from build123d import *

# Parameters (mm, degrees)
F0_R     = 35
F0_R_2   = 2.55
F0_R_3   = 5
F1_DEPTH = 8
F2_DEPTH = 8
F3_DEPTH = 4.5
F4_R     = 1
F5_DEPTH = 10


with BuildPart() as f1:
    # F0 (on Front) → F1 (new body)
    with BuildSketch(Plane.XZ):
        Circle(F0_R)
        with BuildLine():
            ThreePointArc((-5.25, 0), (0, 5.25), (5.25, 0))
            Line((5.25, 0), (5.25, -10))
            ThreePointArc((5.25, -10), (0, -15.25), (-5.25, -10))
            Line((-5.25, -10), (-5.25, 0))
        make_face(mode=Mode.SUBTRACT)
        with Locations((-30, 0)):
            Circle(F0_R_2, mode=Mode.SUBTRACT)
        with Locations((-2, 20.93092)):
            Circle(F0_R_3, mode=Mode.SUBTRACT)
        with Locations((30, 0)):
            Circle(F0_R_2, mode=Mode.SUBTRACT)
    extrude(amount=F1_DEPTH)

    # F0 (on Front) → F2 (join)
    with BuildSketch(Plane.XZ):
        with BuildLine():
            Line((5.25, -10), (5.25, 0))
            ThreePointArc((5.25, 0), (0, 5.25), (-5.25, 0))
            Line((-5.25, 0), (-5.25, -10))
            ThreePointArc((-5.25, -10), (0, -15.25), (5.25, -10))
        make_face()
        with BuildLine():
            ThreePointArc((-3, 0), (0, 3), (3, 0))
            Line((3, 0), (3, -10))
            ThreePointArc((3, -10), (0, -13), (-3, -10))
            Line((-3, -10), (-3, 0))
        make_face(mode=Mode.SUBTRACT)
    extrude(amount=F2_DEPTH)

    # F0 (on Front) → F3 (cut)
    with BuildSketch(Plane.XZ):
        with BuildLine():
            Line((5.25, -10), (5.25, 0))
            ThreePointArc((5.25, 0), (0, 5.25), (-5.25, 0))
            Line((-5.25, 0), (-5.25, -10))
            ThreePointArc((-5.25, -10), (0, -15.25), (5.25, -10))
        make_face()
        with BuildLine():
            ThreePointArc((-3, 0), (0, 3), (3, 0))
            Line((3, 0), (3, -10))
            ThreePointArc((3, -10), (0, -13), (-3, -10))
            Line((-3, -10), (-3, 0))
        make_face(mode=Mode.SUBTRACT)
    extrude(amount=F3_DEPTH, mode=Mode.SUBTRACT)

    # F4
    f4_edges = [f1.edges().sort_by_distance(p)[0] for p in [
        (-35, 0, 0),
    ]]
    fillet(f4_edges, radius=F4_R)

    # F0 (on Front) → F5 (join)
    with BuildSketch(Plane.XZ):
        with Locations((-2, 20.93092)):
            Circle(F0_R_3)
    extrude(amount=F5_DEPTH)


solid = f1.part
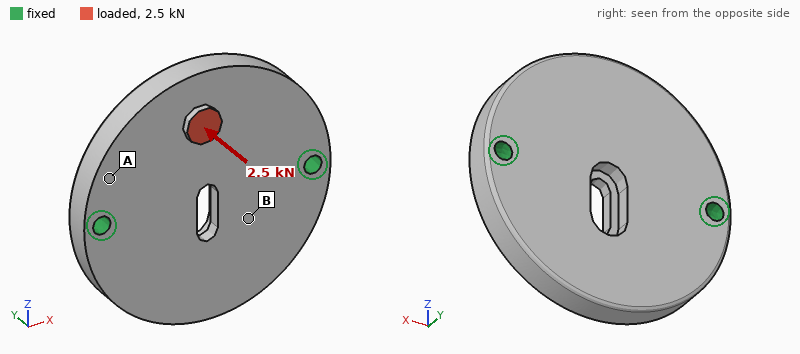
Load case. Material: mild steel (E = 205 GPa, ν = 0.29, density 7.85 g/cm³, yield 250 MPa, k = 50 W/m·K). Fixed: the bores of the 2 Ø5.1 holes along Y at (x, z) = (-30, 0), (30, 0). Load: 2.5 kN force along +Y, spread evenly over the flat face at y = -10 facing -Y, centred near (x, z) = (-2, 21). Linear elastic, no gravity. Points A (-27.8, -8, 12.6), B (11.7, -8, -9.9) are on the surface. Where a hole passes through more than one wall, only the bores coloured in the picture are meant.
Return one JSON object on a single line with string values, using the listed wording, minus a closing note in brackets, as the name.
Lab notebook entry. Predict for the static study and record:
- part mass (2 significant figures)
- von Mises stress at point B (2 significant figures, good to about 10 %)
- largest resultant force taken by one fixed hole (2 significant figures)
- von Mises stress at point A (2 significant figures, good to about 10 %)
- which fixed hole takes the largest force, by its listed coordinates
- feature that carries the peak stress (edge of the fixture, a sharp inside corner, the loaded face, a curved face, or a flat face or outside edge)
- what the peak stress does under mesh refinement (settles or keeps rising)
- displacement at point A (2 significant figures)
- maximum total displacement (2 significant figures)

{"part mass": "230 g", "von Mises stress at point B": "23 MPa", "largest resultant force taken by one fixed hole": "1.4 kN", "von Mises stress at point A": "61 MPa", "which fixed hole takes the largest force, by its listed coordinates": "(-30, 0)", "feature that carries the peak stress": "edge of the fixture", "what the peak stress does under mesh refinement": "keeps rising", "displacement at point A": "13 µm", "maximum total displacement": "69 µm"}
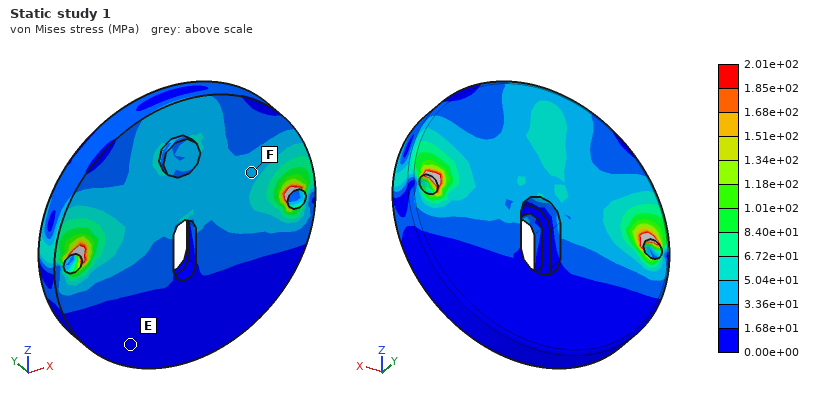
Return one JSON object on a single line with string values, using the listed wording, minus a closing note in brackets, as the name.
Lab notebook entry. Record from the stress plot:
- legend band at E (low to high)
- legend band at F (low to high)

{"legend band at E": "0.00e+00 to 1.68e+01 MPa", "legend band at F": "3.36e+01 to 5.04e+01 MPa"}
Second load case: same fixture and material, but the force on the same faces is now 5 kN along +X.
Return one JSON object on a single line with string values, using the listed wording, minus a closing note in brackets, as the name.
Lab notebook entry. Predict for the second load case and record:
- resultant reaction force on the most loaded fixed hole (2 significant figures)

{"resultant reaction force on the most loaded fixed hole": "3.1 kN"}
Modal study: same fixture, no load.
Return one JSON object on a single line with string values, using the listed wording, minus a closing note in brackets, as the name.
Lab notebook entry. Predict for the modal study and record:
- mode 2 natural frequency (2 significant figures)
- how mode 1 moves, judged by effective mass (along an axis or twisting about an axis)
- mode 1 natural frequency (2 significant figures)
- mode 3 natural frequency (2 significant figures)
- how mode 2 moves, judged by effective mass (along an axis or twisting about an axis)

{"mode 2 natural frequency": "5400 Hz", "how mode 1 moves, judged by effective mass": "twisting about X", "mode 1 natural frequency": "4100 Hz", "mode 3 natural frequency": "12 kHz", "how mode 2 moves, judged by effective mass": "along Y"}
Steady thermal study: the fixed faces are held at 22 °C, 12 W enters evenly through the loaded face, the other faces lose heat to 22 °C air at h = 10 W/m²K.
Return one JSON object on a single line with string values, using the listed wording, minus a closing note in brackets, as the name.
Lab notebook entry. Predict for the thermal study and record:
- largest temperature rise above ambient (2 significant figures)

{"largest temperature rise above ambient": "32 K"}
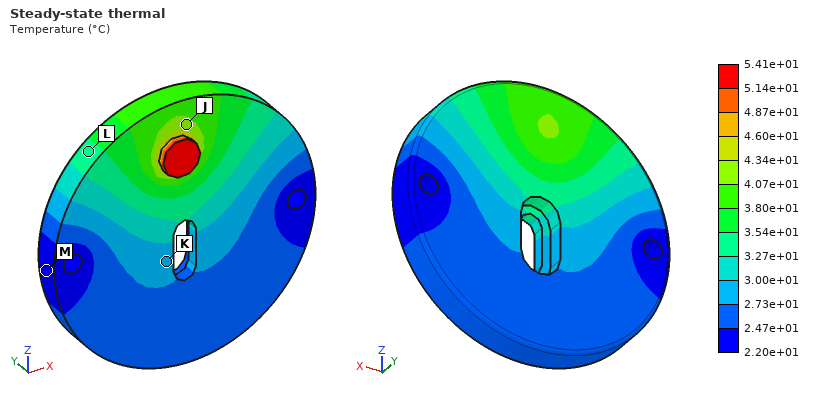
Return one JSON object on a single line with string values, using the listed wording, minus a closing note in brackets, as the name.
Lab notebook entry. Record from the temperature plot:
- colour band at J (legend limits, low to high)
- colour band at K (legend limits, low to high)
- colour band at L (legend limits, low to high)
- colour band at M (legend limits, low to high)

{"colour band at J": "4.07e+01 to 4.34e+01 °C", "colour band at K": "2.73e+01 to 3.00e+01 °C", "colour band at L": "3.27e+01 to 3.54e+01 °C", "colour band at M": "2.20e+01 to 2.47e+01 °C"}
